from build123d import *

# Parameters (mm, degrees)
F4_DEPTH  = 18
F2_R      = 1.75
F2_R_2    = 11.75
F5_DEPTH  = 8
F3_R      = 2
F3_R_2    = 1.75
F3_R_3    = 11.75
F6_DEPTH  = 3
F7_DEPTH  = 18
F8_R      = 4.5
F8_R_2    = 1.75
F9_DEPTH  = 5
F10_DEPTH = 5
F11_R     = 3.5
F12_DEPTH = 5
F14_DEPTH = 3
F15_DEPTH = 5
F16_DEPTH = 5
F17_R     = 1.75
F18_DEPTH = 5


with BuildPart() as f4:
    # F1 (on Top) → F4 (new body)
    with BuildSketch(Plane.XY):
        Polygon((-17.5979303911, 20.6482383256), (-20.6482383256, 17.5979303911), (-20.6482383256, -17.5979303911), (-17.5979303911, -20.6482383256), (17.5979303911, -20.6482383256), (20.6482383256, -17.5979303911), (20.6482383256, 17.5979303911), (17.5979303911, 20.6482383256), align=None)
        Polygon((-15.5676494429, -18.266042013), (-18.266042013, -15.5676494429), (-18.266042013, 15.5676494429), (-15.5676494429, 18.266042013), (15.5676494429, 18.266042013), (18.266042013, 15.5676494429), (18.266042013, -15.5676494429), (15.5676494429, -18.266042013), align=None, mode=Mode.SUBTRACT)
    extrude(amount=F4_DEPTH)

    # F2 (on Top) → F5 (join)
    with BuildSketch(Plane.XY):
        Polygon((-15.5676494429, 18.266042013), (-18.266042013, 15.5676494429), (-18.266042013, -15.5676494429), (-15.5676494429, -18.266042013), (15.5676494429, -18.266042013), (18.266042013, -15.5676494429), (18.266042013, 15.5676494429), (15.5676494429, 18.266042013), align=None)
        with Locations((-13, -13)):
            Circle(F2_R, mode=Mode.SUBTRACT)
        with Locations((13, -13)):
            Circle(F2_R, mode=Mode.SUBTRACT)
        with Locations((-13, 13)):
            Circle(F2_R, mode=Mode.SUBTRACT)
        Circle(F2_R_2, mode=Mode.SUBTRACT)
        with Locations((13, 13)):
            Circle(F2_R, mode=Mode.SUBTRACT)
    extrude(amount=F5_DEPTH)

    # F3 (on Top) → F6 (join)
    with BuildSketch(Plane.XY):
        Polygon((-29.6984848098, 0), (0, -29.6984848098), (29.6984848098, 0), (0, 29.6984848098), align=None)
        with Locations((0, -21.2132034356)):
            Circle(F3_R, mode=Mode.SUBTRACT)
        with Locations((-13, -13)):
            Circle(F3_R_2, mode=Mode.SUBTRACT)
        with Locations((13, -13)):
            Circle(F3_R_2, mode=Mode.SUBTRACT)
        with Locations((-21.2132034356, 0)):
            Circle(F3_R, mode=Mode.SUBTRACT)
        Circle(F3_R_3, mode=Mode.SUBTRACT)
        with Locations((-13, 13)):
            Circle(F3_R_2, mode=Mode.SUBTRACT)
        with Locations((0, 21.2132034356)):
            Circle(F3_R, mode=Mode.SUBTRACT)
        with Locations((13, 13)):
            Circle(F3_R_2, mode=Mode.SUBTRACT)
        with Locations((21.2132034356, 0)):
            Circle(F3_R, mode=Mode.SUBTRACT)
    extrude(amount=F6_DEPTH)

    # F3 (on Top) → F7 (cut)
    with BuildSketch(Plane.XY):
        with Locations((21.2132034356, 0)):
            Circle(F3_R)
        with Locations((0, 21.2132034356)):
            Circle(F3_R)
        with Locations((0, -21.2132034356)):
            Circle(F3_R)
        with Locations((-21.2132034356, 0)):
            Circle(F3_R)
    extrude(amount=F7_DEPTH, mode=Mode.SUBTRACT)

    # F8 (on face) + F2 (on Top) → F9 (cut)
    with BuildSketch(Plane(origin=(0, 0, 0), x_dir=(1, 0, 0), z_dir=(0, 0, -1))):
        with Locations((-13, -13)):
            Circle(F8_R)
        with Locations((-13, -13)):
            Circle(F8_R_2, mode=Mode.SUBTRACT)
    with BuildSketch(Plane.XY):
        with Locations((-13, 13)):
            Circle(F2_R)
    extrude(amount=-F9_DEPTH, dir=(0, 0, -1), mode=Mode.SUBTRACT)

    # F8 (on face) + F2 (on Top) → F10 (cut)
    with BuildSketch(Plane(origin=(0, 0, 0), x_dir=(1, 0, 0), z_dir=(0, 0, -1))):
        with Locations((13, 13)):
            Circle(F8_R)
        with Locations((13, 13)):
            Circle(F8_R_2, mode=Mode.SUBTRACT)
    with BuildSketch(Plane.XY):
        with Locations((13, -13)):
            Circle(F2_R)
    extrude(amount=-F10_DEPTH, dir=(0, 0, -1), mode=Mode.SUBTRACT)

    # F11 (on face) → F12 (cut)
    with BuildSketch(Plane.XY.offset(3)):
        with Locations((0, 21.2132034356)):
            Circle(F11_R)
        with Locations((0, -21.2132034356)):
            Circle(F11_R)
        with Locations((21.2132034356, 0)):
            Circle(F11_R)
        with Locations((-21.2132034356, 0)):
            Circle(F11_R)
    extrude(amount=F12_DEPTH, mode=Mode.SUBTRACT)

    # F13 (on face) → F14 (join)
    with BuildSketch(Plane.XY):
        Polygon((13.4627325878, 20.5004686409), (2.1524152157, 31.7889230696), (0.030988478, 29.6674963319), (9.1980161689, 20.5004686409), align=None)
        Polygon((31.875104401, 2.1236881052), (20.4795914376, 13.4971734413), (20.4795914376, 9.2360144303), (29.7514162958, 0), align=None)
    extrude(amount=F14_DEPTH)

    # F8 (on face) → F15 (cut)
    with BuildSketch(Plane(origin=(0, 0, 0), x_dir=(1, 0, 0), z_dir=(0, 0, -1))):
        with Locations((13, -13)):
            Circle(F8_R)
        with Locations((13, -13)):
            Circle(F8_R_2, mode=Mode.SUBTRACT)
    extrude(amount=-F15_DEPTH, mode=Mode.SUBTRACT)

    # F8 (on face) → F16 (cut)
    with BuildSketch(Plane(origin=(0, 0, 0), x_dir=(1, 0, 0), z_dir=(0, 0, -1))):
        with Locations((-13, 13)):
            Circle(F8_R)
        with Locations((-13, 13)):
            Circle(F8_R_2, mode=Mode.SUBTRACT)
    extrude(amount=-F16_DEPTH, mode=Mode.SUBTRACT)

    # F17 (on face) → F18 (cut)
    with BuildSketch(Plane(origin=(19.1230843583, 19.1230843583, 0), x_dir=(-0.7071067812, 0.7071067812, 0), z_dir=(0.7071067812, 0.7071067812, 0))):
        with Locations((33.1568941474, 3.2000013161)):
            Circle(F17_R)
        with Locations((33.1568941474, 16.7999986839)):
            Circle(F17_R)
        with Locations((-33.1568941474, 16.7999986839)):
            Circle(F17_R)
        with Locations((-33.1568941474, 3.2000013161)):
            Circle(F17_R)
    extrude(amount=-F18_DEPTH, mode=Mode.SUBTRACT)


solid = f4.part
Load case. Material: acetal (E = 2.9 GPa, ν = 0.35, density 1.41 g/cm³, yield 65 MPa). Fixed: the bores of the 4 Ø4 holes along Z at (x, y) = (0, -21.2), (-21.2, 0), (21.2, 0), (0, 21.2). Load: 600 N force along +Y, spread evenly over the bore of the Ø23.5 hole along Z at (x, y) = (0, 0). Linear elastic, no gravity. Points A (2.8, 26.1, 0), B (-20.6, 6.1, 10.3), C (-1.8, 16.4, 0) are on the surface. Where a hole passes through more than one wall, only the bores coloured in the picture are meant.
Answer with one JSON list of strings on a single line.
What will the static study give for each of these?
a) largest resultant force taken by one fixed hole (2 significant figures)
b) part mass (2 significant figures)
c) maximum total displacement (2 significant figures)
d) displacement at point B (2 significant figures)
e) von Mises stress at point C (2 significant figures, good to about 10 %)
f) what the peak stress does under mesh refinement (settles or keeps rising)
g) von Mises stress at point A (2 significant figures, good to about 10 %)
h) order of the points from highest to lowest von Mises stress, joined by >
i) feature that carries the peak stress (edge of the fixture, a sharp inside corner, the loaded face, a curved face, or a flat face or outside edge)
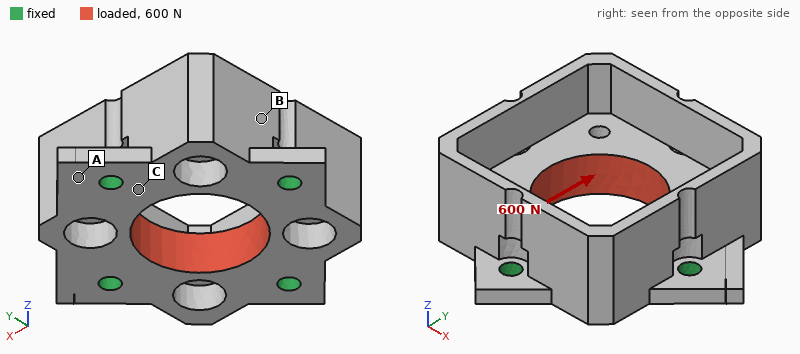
["170 N", "18 g", "29 µm", "14 µm", "3.0 MPa", "keeps rising", "1.6 MPa", "C > A > B", "edge of the fixture"]
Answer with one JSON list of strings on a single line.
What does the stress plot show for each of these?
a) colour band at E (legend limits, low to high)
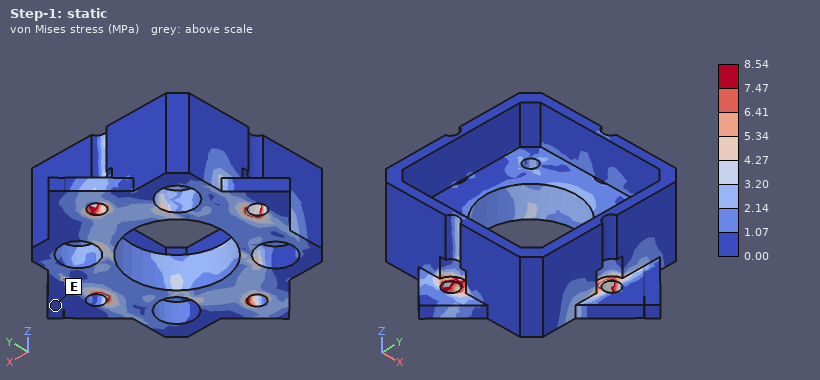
["0.00 to 1.07 MPa"]
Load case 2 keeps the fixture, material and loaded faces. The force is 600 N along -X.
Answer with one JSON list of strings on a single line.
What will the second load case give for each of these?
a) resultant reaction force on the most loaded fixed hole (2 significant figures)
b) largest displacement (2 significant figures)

["170 N", "30 µm"]
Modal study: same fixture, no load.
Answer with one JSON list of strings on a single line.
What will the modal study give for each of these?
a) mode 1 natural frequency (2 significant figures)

["3000 Hz"]
